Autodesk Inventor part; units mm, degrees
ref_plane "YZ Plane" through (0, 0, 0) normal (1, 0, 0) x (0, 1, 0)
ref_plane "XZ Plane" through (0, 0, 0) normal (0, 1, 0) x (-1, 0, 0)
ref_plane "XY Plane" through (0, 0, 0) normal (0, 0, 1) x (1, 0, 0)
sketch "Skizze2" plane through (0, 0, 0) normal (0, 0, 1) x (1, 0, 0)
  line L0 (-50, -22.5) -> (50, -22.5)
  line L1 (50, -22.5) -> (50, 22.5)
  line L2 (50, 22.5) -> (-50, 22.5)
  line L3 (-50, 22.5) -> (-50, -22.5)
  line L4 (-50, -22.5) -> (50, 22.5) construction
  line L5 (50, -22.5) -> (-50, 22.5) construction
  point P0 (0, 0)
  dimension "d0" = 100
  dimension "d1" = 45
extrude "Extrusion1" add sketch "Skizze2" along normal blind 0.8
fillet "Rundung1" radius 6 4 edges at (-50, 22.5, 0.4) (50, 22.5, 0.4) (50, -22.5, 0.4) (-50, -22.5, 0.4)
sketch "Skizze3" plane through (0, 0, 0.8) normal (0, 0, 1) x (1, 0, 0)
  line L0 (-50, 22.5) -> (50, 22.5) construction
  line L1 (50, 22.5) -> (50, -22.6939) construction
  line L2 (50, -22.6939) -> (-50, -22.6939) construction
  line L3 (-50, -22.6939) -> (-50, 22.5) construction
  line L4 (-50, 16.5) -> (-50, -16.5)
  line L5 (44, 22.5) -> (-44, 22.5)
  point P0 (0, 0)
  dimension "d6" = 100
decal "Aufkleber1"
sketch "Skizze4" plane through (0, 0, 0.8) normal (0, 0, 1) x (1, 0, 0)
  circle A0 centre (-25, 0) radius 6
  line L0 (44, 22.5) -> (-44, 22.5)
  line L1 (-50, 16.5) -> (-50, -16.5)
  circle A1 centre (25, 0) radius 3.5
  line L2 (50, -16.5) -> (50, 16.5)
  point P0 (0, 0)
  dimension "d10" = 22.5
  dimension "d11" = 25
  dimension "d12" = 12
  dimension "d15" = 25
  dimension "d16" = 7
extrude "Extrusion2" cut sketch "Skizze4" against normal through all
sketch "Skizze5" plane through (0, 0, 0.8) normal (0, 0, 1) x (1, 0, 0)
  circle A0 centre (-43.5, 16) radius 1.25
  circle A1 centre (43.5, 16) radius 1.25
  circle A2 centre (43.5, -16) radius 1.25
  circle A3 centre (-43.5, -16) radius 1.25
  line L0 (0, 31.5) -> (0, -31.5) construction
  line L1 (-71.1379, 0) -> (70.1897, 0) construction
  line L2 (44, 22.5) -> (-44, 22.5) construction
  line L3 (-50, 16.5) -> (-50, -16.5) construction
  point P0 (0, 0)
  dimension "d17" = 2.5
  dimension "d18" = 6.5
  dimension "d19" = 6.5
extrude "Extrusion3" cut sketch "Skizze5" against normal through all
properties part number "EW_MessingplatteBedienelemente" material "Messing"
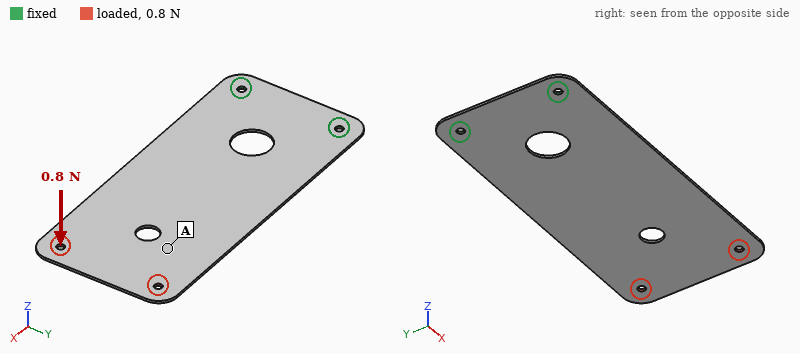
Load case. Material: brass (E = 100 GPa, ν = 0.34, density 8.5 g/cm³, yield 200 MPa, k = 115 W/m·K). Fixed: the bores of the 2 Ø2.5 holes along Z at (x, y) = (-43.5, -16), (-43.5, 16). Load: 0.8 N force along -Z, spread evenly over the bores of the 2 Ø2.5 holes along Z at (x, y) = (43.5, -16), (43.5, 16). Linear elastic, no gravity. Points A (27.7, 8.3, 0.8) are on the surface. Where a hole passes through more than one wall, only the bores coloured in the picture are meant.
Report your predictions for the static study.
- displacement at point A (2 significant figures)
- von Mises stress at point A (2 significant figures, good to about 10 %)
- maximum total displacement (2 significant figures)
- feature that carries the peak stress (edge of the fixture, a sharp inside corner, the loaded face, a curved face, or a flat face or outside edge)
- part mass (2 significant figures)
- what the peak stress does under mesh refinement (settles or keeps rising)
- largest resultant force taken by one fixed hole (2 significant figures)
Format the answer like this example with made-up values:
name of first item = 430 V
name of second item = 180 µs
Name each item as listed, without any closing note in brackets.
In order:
displacement at point A = 0.76 mm
von Mises stress at point A = 3.2 MPa
maximum total displacement = 1.1 mm
feature that carries the peak stress = edge of the fixture
part mass = 29 g
what the peak stress does under mesh refinement = keeps rising
largest resultant force taken by one fixed hole = 0.40 N
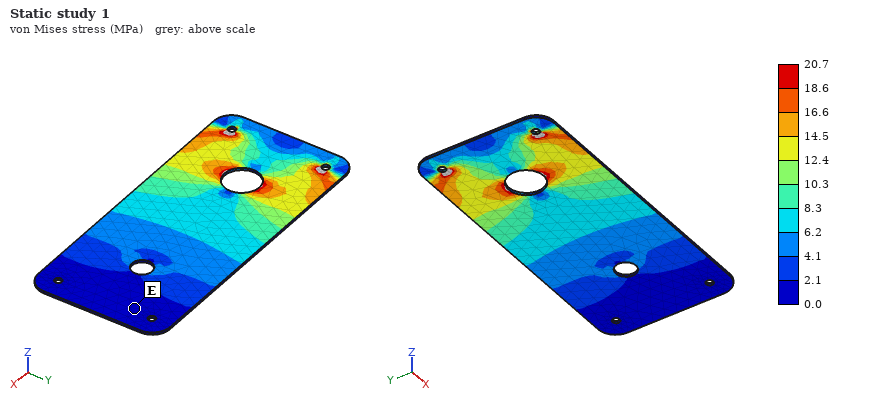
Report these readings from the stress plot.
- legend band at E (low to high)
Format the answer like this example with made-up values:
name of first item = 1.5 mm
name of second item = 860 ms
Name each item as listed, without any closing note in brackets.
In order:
legend band at E = 0.0 to 2.1 MPa
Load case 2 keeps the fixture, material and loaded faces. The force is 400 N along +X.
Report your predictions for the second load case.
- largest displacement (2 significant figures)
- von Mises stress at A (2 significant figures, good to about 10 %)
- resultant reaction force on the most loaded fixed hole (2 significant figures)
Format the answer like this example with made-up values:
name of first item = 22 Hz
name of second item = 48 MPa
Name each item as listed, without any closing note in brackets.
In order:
largest displacement = 14 µm
von Mises stress at A = 11 MPa
resultant reaction force on the most loaded fixed hole = 200 N
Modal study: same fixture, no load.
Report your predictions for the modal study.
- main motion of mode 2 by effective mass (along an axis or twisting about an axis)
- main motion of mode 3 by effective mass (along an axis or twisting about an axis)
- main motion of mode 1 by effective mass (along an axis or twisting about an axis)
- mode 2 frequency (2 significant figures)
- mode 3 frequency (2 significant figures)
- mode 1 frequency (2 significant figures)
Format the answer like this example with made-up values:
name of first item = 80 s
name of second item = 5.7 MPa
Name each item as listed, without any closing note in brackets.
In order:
main motion of mode 2 by effective mass = twisting about X
main motion of mode 3 by effective mass = along Z
main motion of mode 1 by effective mass = along Z
mode 2 frequency = 230 Hz
mode 3 frequency = 320 Hz
mode 1 frequency = 48 Hz
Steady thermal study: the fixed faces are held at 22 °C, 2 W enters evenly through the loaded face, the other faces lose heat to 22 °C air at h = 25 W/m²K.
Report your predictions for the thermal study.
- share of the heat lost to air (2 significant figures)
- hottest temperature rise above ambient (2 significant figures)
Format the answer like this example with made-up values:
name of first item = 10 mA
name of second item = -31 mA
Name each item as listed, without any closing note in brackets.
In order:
share of the heat lost to air = 81 %
hottest temperature rise above ambient = 21 K
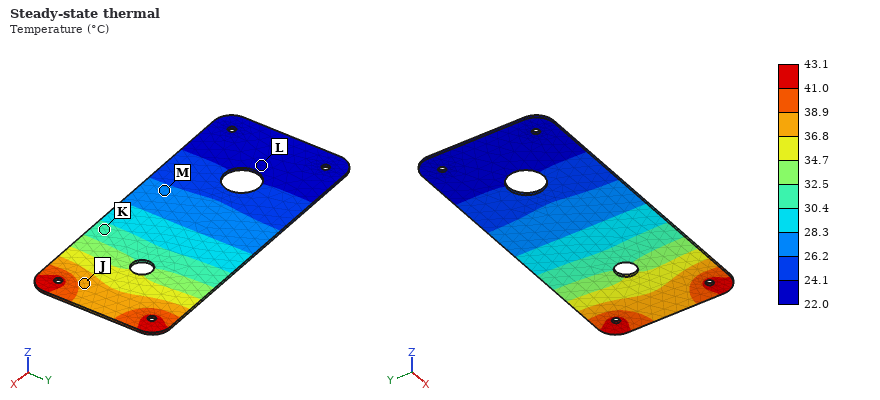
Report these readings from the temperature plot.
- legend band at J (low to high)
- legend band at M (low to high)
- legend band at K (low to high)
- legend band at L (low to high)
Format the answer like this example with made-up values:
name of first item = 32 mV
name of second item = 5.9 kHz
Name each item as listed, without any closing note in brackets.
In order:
legend band at J = 36.8 to 38.9 °C
legend band at M = 26.2 to 28.3 °C
legend band at K = 30.4 to 32.5 °C
legend band at L = 22.0 to 24.1 °C
